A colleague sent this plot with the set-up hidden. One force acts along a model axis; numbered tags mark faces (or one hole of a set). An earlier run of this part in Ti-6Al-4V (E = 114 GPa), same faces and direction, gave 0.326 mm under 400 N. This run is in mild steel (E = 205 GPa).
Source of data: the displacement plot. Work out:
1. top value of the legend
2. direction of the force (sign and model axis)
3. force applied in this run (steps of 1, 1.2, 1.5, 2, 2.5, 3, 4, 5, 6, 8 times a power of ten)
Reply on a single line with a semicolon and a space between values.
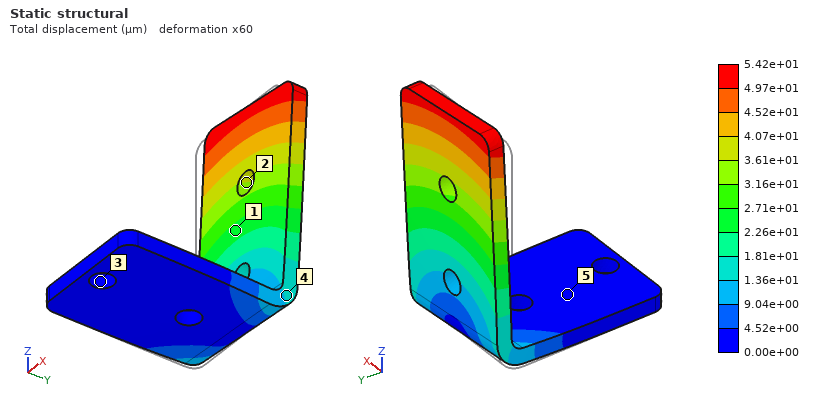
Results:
5.42e+01 µm; +X; 120 N
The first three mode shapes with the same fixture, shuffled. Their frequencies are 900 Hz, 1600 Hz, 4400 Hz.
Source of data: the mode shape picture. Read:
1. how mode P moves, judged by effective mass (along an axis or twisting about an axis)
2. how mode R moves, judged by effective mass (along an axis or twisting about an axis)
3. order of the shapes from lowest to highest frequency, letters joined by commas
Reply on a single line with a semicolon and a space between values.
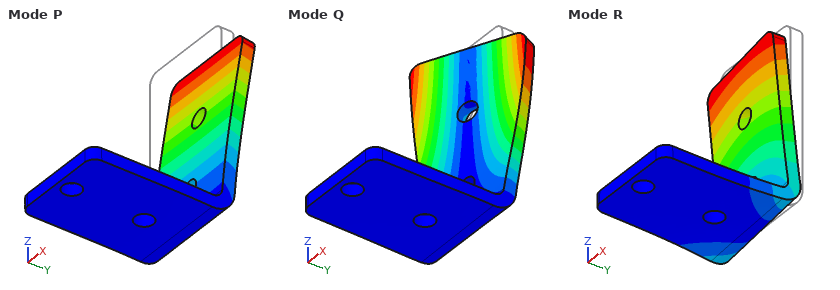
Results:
along Y; along X; P, R, Q
